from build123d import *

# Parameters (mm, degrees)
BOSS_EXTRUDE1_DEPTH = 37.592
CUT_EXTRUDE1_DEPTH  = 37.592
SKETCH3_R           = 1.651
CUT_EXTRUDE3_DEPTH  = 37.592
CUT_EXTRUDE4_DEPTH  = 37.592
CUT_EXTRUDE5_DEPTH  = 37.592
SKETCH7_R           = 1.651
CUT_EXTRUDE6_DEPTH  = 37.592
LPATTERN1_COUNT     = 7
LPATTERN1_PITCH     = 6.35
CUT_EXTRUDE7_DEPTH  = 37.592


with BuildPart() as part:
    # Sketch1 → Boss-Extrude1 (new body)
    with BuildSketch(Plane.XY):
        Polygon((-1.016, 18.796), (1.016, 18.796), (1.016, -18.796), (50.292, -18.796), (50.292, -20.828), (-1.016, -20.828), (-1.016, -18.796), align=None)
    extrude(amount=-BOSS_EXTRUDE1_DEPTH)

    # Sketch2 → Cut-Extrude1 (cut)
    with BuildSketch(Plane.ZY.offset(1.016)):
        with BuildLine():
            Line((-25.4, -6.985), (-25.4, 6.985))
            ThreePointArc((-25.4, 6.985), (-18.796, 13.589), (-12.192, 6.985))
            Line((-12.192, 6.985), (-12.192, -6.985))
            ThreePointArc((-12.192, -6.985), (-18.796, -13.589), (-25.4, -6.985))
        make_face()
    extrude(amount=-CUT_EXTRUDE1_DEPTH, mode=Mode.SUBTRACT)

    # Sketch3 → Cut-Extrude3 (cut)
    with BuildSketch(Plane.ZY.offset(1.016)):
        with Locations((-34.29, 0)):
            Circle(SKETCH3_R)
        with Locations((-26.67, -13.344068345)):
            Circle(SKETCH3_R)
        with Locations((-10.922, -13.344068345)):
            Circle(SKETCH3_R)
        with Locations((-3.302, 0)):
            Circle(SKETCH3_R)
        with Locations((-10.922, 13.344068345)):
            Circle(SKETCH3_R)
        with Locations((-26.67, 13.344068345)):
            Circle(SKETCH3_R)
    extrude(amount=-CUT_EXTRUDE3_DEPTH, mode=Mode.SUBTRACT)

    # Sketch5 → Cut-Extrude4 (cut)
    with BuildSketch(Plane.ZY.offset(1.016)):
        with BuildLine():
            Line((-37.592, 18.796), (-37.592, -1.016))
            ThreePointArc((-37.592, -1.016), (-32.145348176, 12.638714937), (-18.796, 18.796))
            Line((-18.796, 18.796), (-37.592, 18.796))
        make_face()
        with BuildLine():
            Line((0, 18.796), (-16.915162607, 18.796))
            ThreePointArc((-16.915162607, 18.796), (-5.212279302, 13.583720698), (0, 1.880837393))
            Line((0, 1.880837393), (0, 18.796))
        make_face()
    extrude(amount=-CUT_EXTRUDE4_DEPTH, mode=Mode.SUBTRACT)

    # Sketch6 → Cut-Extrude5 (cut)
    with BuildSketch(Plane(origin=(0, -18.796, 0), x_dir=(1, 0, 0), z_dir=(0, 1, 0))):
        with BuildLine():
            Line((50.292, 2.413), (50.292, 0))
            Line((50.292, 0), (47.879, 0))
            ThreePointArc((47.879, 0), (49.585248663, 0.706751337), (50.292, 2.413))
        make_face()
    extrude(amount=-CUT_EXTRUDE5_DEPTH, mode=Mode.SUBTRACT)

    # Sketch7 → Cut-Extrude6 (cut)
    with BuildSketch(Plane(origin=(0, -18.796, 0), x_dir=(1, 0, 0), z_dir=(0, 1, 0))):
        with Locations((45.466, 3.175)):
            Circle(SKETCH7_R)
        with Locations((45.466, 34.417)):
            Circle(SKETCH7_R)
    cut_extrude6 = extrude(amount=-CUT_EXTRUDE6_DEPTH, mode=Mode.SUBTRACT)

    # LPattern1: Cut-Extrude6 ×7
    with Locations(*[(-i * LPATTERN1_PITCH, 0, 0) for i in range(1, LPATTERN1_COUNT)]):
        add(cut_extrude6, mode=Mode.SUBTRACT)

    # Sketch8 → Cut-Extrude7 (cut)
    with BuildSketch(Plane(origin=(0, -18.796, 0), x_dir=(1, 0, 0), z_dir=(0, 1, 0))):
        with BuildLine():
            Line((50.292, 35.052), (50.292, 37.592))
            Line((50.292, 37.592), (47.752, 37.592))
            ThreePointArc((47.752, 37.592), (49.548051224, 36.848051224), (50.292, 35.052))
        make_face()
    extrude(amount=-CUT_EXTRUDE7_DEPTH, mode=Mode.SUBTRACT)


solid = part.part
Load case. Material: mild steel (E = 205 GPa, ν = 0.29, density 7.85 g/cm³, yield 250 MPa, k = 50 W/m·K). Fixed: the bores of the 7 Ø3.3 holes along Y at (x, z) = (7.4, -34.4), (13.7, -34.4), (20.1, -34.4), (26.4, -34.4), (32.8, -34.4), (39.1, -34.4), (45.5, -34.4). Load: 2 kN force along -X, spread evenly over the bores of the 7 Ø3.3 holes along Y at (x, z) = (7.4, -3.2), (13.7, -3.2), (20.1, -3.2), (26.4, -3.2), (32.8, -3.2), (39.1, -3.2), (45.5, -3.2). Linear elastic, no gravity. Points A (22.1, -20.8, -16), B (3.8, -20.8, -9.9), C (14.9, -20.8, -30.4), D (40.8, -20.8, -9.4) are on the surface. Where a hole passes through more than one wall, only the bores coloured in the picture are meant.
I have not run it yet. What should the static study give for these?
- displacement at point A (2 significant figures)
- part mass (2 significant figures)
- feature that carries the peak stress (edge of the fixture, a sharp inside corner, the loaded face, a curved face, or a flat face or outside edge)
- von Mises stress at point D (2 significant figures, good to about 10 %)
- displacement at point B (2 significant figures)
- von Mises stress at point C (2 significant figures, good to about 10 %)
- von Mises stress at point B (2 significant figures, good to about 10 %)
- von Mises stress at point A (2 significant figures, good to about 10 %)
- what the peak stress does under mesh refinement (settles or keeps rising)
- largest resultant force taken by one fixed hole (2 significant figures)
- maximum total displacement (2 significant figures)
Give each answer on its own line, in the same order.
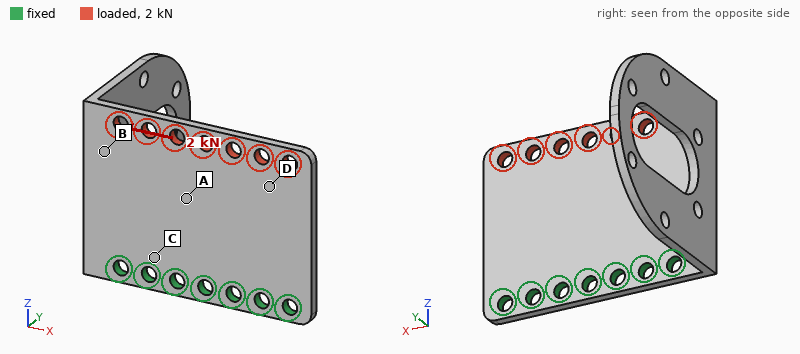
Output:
7.5 µm
43 g
edge of the fixture
34 MPa
12 µm
58 MPa
18 MPa
50 MPa
keeps rising
1.3 kN
18 µm
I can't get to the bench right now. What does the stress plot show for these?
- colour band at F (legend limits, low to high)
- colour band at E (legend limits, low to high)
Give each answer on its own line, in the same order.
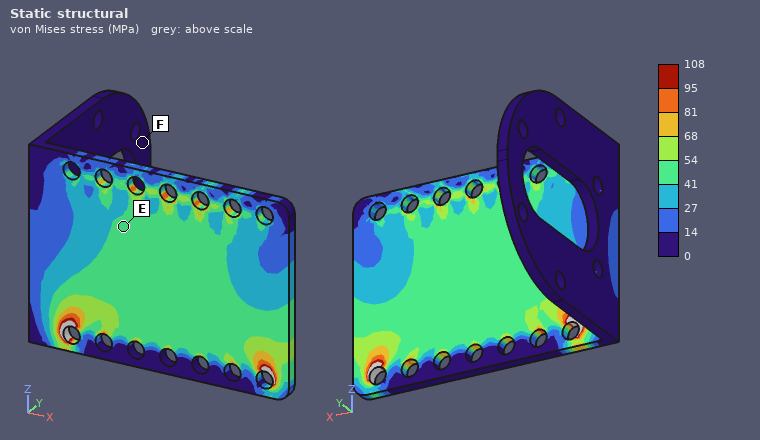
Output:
0 to 14 MPa
41 to 54 MPa
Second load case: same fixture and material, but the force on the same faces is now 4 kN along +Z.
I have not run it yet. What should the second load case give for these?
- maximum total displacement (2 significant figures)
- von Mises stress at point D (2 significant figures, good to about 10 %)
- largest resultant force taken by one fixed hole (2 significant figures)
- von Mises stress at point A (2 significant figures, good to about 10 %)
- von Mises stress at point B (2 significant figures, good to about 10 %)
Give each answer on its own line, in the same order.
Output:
7.5 µm
45 MPa
760 N
46 MPa
23 MPa
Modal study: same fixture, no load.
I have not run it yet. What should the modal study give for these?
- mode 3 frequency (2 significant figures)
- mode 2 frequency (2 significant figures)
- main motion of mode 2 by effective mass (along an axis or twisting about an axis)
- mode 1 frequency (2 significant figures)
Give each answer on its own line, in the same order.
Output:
2200 Hz
1200 Hz
along Y
920 Hz
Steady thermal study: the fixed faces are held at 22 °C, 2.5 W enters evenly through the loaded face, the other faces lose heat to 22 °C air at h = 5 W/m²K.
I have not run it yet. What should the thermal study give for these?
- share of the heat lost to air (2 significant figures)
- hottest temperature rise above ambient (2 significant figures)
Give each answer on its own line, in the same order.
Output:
7.3 %
16 K
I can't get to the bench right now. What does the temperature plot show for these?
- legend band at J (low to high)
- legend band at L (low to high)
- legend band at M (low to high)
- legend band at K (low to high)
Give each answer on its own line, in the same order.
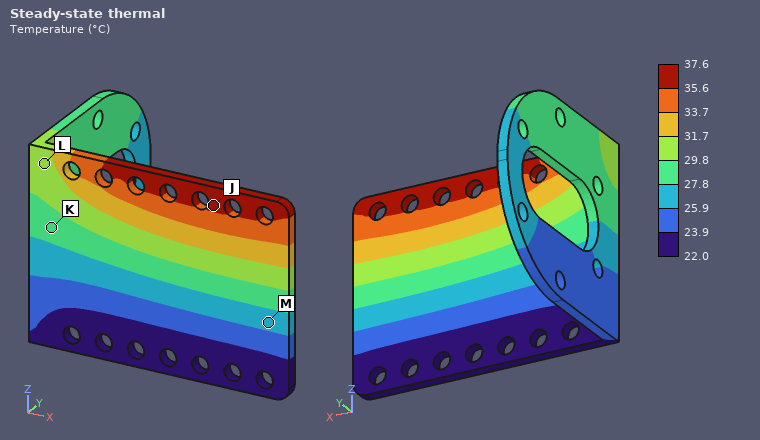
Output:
35.6 to 37.6 °C
29.8 to 31.7 °C
25.9 to 27.8 °C
27.8 to 29.8 °C
